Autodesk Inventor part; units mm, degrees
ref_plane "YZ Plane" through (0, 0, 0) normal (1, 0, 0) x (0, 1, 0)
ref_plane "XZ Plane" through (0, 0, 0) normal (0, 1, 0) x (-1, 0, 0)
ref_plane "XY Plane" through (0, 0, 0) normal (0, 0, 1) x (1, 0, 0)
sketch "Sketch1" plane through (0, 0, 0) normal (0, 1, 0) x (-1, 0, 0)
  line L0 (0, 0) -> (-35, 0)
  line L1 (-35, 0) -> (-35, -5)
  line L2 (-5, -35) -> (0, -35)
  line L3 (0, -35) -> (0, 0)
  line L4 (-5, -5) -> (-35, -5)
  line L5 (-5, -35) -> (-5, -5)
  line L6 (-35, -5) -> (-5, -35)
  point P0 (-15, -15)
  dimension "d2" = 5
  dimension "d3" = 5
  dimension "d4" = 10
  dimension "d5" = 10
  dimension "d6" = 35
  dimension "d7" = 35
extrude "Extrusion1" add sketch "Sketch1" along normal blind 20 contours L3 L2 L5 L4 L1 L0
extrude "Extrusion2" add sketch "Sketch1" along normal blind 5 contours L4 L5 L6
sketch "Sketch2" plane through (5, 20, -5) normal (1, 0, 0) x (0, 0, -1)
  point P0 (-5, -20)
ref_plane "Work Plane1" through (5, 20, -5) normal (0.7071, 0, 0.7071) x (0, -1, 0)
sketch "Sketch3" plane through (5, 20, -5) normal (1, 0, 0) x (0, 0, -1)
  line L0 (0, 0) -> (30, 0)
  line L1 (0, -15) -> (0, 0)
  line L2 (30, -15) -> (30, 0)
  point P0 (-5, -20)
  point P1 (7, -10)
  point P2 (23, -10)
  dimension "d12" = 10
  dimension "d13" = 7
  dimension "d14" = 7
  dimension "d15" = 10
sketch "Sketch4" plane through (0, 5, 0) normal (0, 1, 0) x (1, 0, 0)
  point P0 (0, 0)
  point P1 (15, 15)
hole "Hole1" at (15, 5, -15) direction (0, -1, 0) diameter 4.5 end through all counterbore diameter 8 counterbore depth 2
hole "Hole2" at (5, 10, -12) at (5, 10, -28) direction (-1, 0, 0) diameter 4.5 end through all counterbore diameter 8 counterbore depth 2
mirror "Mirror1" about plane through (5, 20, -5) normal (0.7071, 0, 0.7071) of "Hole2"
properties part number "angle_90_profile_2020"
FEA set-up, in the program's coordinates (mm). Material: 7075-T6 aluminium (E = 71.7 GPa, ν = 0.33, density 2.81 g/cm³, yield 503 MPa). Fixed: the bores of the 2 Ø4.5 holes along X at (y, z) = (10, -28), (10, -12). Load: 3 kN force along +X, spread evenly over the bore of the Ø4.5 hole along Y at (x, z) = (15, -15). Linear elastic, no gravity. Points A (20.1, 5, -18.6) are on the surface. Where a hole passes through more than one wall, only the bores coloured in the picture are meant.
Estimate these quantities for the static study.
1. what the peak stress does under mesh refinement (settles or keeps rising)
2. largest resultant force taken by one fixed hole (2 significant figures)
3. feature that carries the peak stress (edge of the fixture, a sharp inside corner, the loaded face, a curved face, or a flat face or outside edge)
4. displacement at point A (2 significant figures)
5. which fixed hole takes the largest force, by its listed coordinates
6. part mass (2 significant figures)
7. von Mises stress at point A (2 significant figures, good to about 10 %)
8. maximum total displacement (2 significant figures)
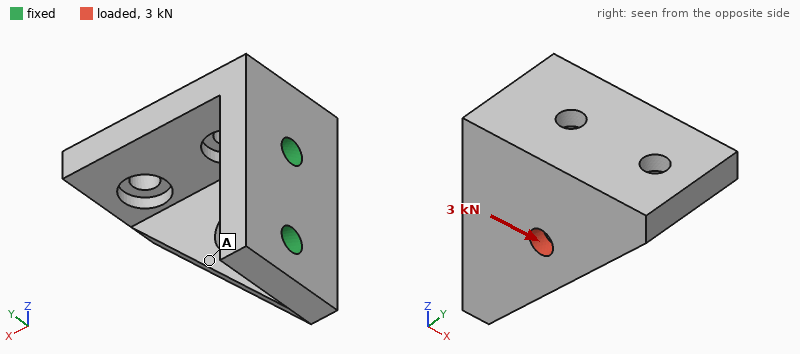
keeps rising
2.3 kN
edge of the fixture
0.14 mm
(10, -12)
23 g
57 MPa
0.25 mm
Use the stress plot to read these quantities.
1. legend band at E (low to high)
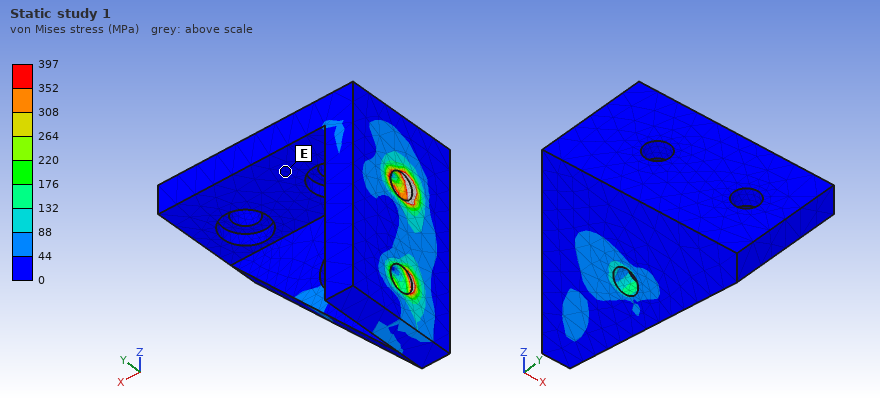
0 to 44 MPa
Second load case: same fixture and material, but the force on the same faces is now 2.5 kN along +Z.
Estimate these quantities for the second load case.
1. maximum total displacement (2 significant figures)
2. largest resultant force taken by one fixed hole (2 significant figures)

0.12 mm
2.5 kN
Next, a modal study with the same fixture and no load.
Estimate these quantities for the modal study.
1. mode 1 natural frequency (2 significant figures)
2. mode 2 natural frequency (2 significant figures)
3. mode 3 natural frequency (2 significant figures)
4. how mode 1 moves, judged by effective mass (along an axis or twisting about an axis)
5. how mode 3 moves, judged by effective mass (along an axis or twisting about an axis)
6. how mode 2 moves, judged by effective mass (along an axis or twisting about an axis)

3400 Hz
5800 Hz
12 kHz
along Y
along X
along Z
